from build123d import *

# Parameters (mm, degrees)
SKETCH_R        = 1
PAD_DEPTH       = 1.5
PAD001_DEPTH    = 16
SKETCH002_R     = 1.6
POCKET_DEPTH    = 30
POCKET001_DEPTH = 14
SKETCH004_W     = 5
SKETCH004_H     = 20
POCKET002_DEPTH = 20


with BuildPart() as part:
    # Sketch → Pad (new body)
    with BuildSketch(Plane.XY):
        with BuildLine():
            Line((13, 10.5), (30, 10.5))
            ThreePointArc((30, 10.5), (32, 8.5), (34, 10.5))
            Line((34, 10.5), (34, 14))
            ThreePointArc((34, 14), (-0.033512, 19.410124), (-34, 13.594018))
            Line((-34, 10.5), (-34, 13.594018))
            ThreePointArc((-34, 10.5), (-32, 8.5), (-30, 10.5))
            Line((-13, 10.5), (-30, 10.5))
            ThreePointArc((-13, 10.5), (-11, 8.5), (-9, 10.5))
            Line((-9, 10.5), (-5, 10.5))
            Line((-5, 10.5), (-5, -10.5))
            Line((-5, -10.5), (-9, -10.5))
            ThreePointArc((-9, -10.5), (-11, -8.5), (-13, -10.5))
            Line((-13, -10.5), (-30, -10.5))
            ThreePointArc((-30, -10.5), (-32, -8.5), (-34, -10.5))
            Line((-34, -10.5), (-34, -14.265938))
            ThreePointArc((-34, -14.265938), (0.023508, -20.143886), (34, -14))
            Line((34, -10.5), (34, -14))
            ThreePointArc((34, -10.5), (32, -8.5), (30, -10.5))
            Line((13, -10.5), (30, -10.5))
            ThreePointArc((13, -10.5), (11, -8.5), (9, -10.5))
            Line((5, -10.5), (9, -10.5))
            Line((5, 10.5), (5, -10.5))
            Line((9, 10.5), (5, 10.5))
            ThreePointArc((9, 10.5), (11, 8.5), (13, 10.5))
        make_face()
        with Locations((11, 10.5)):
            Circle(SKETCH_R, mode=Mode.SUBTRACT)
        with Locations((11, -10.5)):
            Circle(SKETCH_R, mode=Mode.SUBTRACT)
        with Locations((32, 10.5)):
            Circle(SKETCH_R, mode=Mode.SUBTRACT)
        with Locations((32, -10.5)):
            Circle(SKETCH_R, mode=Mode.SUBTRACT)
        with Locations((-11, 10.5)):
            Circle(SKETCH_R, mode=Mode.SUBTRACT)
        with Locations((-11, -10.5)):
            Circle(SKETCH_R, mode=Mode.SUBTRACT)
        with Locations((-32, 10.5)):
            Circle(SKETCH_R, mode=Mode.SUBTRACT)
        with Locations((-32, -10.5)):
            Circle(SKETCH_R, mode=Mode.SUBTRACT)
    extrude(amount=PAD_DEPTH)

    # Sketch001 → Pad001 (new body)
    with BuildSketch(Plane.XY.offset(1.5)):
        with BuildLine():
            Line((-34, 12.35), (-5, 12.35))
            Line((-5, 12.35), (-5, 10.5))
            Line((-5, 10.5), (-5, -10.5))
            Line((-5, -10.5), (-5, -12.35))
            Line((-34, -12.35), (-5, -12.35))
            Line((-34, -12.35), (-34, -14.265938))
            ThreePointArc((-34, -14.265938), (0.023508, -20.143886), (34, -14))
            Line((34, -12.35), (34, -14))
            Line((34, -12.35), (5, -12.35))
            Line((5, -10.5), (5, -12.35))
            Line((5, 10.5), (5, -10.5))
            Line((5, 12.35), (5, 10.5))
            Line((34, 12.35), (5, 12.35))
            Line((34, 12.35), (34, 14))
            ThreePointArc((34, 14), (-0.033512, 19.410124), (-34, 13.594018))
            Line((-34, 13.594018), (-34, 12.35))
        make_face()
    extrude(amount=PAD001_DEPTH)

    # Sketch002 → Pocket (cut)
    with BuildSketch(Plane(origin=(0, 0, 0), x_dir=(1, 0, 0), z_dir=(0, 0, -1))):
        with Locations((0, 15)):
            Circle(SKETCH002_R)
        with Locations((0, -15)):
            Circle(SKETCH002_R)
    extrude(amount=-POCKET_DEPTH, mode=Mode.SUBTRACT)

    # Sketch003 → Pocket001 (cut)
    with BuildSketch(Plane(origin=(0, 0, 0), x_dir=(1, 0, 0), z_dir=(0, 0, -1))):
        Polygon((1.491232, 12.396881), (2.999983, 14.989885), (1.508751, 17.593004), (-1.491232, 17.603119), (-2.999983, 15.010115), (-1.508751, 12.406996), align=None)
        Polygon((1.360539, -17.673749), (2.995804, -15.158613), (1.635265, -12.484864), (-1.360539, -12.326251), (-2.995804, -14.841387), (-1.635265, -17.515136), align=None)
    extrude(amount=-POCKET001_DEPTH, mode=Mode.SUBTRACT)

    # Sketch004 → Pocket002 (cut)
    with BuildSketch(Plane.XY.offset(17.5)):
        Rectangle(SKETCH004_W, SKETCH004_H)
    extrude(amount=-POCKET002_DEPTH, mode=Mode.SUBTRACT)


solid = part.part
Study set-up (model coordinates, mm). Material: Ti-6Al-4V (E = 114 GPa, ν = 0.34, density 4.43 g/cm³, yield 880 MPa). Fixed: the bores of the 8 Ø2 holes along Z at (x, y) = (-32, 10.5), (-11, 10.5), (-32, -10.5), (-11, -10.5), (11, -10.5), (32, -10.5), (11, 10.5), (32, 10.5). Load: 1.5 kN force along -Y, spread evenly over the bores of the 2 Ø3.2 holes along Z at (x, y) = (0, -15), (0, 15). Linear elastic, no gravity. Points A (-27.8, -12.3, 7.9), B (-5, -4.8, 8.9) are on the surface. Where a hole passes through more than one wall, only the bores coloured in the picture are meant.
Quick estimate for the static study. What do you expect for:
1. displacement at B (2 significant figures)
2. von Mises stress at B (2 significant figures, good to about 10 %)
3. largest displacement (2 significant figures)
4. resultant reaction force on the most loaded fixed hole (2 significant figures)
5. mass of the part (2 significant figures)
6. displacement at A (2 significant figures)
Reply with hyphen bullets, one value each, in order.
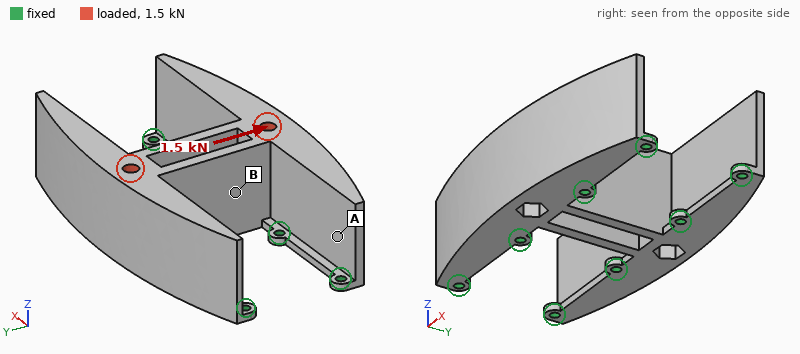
- 15 µm
- 26 MPa
- 32 µm
- 550 N
- 68 g
- 11 µm
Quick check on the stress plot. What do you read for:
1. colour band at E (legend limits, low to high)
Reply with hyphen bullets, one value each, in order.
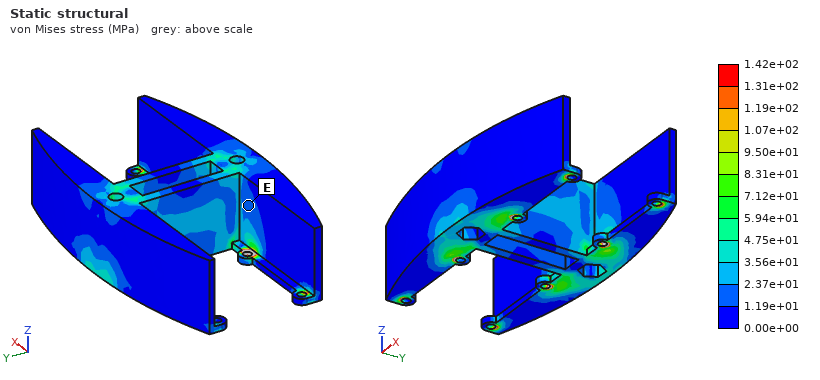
- 1.19e+01 to 2.37e+01 MPa
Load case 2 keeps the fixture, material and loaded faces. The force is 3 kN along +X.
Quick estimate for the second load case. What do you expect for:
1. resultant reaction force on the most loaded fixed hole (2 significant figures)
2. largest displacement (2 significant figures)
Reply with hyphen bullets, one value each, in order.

- 490 N
- 13 µm
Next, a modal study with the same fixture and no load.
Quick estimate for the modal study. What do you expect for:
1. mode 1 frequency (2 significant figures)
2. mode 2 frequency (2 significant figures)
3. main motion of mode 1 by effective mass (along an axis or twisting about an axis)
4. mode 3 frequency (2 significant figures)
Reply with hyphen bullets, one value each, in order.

- 5900 Hz
- 9600 Hz
- along Y
- 9900 Hz
